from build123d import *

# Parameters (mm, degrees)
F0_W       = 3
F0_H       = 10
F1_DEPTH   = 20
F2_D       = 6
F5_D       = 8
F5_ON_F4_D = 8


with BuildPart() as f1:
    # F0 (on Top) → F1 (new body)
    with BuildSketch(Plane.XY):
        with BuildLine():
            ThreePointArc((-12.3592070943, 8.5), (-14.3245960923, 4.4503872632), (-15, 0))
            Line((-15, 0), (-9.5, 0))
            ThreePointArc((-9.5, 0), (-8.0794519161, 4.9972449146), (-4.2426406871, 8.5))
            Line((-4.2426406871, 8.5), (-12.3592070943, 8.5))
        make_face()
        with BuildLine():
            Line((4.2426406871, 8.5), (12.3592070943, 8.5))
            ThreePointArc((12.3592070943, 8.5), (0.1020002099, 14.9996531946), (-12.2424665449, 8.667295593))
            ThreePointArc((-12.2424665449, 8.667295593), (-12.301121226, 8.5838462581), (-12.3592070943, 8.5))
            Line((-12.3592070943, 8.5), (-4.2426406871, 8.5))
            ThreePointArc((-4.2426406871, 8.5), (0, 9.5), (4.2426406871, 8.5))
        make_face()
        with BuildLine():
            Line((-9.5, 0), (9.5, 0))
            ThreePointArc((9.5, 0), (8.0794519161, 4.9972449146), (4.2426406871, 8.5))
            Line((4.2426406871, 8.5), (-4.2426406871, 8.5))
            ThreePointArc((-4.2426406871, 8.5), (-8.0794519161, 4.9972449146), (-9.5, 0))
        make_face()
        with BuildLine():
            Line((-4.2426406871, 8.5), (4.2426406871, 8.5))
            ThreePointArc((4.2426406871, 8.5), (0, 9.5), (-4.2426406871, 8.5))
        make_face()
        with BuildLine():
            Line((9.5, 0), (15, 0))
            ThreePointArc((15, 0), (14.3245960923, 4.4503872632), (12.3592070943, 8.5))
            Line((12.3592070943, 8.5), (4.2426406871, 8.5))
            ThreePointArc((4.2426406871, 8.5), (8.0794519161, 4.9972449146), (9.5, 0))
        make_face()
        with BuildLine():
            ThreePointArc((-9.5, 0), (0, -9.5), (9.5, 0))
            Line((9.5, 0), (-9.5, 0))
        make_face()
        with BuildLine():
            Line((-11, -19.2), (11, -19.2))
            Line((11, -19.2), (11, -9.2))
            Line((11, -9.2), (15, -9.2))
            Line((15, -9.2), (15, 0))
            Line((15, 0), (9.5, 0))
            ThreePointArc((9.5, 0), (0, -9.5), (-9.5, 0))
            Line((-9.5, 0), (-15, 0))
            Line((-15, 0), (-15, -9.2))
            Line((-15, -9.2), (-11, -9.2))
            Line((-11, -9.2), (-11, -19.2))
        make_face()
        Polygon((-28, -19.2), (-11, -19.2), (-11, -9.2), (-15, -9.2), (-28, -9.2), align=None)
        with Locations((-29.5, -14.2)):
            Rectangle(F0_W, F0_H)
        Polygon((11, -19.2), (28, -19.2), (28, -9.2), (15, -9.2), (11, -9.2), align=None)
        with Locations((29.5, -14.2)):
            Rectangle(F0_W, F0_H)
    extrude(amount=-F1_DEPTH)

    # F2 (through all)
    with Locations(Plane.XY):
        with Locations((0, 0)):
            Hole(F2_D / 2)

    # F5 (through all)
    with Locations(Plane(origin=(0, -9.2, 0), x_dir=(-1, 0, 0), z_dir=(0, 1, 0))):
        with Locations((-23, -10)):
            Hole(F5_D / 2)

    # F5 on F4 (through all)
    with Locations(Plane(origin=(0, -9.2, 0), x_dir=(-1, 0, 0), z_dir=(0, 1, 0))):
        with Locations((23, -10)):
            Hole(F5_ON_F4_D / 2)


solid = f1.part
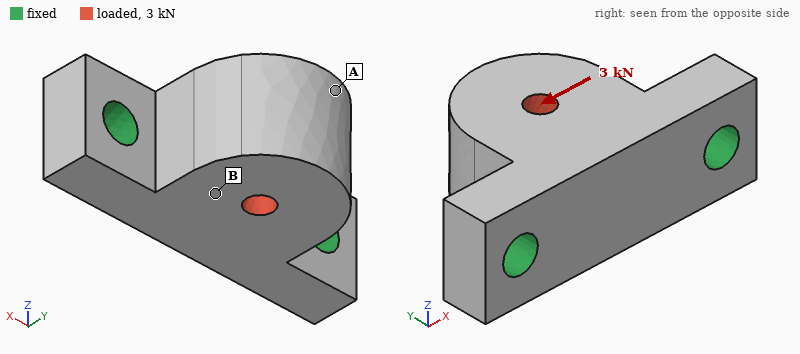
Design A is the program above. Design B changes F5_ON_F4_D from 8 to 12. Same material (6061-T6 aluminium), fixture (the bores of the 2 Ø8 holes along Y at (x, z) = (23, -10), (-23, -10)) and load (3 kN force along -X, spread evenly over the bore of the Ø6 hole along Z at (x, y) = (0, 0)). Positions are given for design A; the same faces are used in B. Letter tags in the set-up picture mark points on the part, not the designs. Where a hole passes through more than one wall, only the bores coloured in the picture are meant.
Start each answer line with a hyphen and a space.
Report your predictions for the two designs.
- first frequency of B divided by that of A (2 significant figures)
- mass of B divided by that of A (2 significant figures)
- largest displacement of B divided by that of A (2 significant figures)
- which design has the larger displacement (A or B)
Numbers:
- 1.1
- 0.97
- 0.91
- A
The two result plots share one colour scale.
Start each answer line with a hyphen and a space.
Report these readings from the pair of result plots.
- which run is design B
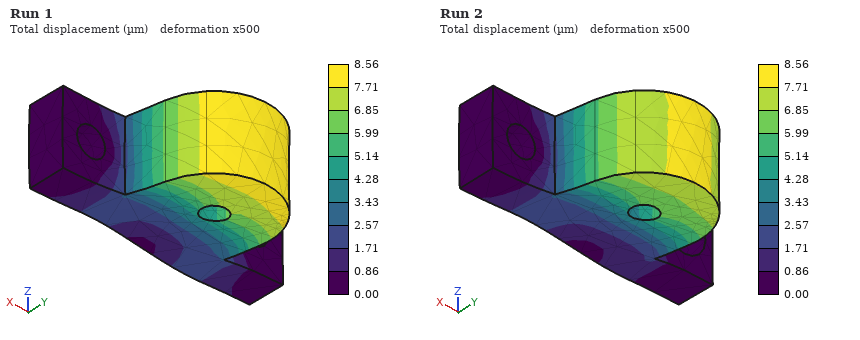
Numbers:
- Run 2
